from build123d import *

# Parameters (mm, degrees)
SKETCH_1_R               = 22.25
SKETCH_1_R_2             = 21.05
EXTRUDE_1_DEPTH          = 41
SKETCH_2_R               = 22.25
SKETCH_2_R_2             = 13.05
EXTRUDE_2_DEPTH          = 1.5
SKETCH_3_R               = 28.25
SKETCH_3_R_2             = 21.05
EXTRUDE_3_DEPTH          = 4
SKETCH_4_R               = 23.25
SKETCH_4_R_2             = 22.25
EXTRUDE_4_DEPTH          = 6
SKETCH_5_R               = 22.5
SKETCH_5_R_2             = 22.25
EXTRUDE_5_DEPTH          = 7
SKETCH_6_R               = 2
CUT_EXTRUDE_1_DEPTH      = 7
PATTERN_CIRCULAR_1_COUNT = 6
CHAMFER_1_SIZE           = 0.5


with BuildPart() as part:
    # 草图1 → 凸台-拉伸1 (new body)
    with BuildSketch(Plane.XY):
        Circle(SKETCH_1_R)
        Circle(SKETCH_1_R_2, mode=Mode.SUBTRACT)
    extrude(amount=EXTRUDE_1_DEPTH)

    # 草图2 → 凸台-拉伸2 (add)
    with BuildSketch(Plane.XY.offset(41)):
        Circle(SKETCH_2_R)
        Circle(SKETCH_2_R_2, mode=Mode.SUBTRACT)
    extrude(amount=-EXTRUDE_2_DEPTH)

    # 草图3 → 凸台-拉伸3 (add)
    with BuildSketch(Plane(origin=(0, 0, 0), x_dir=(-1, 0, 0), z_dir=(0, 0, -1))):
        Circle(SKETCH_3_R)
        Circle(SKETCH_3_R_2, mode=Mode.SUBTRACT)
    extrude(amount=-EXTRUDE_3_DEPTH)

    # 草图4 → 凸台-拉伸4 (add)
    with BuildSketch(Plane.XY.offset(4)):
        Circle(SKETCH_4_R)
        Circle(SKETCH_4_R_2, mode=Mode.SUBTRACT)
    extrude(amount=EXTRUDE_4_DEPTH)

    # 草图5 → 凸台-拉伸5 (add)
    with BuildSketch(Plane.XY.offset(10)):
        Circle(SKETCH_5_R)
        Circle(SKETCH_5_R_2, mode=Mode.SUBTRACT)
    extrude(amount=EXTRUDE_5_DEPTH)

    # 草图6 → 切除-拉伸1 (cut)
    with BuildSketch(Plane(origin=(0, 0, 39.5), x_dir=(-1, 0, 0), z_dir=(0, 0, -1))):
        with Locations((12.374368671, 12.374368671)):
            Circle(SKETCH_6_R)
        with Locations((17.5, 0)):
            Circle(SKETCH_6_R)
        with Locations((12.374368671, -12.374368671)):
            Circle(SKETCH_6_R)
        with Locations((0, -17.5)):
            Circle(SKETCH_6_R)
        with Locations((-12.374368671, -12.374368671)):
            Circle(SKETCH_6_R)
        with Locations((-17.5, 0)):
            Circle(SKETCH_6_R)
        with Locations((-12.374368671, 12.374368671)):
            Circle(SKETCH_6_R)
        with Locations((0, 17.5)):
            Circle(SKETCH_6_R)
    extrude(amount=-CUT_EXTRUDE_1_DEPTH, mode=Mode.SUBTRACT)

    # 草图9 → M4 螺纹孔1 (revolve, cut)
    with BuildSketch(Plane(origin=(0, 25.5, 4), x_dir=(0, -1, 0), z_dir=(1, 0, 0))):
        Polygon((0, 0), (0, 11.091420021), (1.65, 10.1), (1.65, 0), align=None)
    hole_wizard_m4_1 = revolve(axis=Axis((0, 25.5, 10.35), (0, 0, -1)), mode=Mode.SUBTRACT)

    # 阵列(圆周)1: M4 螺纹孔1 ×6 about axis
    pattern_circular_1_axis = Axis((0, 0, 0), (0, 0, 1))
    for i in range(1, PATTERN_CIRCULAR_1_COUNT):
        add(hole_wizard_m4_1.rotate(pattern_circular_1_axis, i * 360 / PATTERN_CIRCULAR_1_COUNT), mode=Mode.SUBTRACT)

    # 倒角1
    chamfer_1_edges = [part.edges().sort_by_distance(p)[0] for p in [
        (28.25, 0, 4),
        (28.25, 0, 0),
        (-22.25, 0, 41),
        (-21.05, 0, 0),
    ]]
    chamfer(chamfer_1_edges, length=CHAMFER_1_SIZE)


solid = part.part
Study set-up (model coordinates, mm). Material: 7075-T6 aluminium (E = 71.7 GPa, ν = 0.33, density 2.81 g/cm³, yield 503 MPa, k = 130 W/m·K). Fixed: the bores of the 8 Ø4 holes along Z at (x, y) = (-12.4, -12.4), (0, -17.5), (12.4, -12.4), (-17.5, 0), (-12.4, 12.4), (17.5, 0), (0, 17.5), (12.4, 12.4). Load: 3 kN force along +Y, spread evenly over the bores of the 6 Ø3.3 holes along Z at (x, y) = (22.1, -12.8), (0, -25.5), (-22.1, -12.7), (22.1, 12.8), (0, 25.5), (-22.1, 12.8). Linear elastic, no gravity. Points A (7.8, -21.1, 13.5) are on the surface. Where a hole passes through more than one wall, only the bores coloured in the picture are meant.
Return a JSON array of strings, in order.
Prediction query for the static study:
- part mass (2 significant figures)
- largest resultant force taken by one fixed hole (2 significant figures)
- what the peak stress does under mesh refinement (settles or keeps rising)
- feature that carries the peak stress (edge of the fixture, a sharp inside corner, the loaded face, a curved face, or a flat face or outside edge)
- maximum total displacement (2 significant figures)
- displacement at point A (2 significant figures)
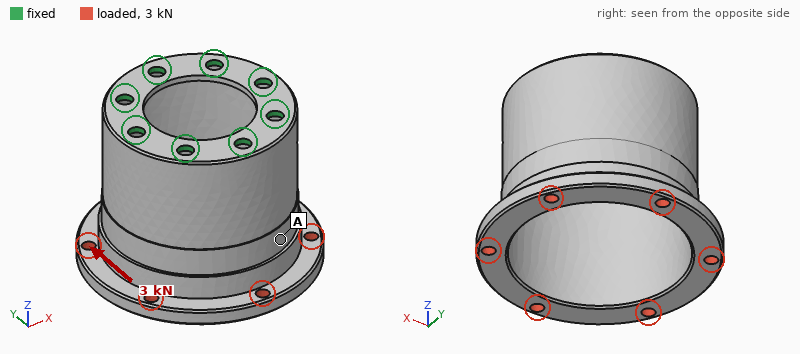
["35 g", "1.4 kN", "keeps rising", "edge of the fixture", "0.18 mm", "0.12 mm"]
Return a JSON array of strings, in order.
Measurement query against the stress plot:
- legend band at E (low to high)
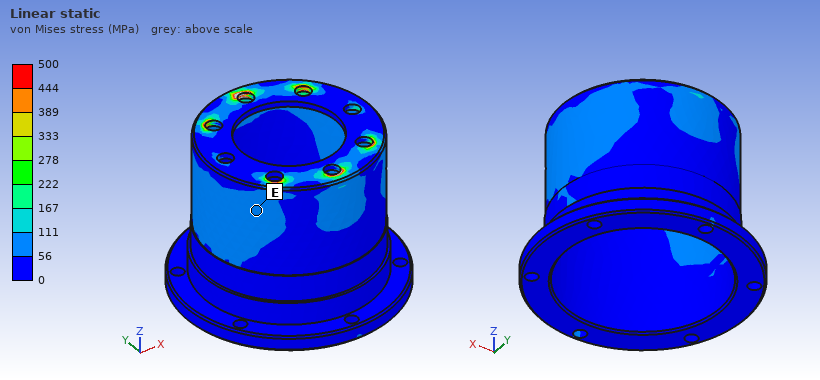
["56 to 111 MPa"]
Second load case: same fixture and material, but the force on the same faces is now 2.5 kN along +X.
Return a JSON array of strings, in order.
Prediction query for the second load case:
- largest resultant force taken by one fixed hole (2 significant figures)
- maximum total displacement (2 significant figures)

["1.1 kN", "0.15 mm"]
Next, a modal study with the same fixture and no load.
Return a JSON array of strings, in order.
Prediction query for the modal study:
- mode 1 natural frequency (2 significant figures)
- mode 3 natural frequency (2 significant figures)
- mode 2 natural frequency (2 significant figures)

["4800 Hz", "5900 Hz", "4800 Hz"]
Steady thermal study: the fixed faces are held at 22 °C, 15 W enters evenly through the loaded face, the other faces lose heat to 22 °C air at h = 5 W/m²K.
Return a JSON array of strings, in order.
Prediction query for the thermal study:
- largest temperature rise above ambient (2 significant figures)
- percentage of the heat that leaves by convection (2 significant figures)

["26 K", "7.0 %"]
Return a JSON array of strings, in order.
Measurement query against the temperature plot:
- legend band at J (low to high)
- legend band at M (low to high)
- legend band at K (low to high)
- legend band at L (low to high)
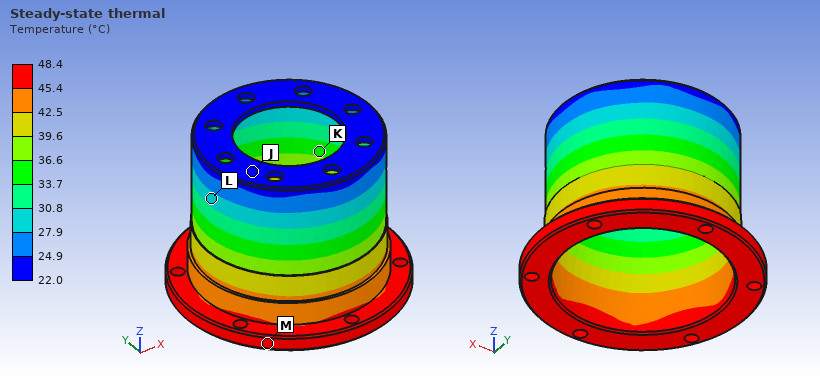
["22.0 to 24.9 °C", "45.4 to 48.4 °C", "33.7 to 36.6 °C", "27.9 to 30.8 °C"]
